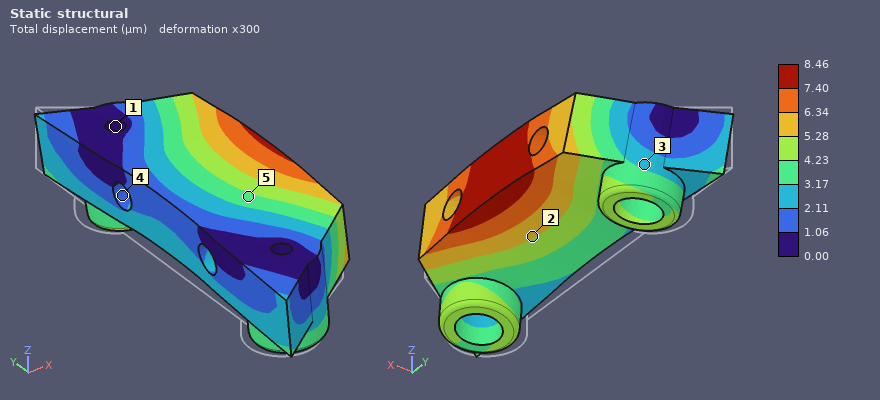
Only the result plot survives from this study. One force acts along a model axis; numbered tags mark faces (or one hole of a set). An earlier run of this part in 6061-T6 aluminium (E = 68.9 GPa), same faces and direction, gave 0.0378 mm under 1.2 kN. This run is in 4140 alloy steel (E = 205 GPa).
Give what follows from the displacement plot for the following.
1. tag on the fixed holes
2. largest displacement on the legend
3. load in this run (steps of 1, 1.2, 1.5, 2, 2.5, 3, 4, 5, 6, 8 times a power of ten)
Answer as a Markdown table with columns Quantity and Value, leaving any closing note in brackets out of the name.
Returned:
| Quantity | Value |
|---|---|
| tag on the fixed holes | 1 |
| largest displacement on the legend | 8.46 µm |
| load in this run | 800 N |
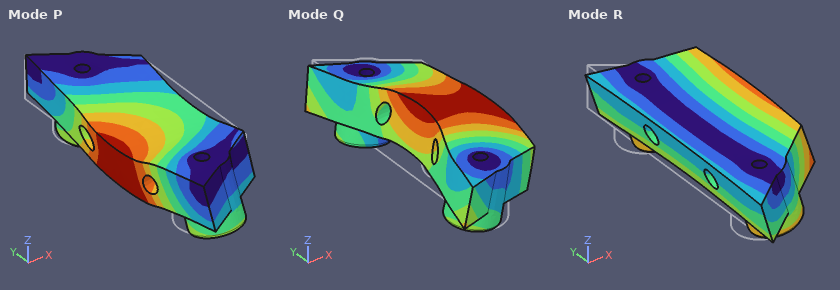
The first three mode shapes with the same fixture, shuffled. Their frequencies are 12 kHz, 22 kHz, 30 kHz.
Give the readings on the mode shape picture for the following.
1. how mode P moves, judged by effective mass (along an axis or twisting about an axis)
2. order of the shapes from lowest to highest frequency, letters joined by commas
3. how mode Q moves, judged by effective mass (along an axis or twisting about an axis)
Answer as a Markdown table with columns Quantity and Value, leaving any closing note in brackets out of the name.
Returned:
| Quantity | Value |
|---|---|
| how mode P moves, judged by effective mass | along Z |
| order of the shapes from lowest to highest frequency, letters joined by commas | R, P, Q |
| how mode Q moves, judged by effective mass | along X |
